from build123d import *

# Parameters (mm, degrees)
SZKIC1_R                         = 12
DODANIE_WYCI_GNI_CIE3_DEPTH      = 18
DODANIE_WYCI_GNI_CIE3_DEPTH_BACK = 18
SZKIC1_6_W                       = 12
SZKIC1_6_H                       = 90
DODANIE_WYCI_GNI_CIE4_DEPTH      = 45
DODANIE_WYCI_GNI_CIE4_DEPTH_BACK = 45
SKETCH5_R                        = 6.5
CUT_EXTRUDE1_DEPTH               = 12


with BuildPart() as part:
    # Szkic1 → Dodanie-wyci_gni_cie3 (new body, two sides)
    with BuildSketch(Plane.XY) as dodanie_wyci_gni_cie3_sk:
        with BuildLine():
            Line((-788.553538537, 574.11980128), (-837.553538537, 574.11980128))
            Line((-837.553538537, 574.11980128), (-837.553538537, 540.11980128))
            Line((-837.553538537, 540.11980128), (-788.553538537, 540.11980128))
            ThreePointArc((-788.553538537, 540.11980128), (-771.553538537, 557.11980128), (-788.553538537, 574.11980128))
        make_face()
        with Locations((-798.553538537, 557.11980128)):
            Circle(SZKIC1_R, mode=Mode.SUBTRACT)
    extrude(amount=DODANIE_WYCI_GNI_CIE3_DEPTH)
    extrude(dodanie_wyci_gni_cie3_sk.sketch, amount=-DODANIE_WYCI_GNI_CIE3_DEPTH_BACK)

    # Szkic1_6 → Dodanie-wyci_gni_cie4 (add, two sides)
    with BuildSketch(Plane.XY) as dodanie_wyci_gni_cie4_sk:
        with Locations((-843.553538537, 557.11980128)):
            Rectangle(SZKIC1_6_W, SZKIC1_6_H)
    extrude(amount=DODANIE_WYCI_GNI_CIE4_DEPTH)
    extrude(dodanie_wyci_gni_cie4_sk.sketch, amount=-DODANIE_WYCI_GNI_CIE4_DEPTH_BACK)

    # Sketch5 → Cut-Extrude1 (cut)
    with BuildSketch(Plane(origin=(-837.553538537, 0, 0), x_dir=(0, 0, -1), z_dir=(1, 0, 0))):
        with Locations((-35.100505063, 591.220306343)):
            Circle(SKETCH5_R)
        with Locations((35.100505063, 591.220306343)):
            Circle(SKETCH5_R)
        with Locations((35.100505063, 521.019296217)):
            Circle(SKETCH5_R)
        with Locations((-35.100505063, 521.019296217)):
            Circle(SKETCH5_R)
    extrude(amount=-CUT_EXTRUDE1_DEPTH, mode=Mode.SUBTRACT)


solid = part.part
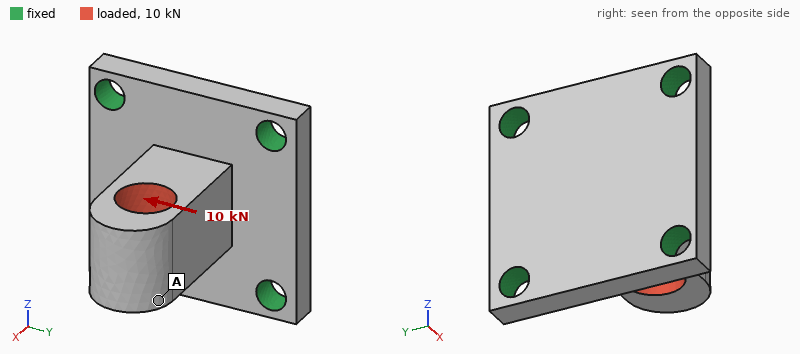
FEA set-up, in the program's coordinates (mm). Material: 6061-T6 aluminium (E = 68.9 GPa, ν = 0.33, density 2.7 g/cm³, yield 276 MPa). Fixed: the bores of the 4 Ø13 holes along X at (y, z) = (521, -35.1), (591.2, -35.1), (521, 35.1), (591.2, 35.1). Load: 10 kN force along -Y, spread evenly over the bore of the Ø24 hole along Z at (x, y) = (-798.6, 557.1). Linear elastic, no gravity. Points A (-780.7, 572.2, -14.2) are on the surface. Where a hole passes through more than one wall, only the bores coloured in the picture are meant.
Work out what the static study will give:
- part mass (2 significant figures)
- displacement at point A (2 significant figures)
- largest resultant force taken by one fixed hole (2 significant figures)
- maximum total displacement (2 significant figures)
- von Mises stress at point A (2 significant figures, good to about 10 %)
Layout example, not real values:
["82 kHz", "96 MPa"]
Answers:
["410 g", "0.22 mm", "4.9 kN", "0.24 mm", "14 MPa"]
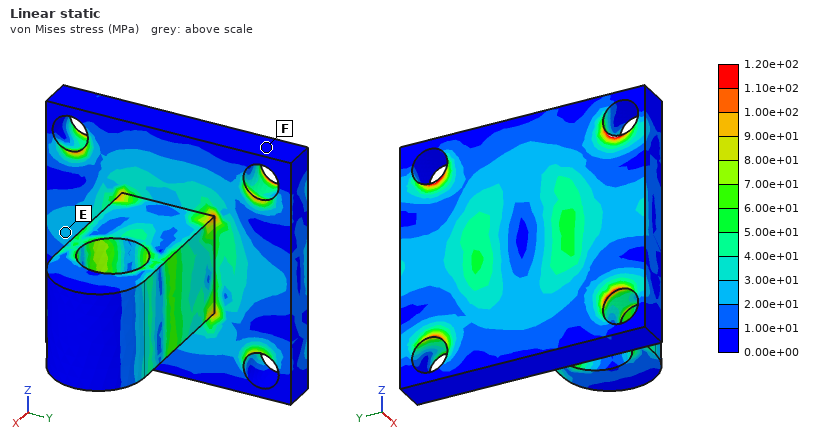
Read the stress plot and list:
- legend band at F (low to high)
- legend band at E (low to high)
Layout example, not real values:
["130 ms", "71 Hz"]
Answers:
["0.00e+00 to 1.00e+01 MPa", "2.00e+01 to 3.00e+01 MPa"]
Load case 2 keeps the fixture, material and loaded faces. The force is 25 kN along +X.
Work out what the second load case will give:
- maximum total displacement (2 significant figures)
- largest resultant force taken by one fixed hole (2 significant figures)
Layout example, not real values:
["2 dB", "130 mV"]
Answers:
["90 µm", "6.6 kN"]
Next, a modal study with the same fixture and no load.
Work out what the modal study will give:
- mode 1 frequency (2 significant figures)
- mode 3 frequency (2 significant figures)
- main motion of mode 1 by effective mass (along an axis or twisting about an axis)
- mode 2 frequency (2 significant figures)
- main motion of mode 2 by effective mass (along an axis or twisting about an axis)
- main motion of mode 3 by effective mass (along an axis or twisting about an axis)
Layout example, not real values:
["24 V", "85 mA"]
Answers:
["3500 Hz", "6200 Hz", "along Y", "3800 Hz", "along Z", "along X"]
